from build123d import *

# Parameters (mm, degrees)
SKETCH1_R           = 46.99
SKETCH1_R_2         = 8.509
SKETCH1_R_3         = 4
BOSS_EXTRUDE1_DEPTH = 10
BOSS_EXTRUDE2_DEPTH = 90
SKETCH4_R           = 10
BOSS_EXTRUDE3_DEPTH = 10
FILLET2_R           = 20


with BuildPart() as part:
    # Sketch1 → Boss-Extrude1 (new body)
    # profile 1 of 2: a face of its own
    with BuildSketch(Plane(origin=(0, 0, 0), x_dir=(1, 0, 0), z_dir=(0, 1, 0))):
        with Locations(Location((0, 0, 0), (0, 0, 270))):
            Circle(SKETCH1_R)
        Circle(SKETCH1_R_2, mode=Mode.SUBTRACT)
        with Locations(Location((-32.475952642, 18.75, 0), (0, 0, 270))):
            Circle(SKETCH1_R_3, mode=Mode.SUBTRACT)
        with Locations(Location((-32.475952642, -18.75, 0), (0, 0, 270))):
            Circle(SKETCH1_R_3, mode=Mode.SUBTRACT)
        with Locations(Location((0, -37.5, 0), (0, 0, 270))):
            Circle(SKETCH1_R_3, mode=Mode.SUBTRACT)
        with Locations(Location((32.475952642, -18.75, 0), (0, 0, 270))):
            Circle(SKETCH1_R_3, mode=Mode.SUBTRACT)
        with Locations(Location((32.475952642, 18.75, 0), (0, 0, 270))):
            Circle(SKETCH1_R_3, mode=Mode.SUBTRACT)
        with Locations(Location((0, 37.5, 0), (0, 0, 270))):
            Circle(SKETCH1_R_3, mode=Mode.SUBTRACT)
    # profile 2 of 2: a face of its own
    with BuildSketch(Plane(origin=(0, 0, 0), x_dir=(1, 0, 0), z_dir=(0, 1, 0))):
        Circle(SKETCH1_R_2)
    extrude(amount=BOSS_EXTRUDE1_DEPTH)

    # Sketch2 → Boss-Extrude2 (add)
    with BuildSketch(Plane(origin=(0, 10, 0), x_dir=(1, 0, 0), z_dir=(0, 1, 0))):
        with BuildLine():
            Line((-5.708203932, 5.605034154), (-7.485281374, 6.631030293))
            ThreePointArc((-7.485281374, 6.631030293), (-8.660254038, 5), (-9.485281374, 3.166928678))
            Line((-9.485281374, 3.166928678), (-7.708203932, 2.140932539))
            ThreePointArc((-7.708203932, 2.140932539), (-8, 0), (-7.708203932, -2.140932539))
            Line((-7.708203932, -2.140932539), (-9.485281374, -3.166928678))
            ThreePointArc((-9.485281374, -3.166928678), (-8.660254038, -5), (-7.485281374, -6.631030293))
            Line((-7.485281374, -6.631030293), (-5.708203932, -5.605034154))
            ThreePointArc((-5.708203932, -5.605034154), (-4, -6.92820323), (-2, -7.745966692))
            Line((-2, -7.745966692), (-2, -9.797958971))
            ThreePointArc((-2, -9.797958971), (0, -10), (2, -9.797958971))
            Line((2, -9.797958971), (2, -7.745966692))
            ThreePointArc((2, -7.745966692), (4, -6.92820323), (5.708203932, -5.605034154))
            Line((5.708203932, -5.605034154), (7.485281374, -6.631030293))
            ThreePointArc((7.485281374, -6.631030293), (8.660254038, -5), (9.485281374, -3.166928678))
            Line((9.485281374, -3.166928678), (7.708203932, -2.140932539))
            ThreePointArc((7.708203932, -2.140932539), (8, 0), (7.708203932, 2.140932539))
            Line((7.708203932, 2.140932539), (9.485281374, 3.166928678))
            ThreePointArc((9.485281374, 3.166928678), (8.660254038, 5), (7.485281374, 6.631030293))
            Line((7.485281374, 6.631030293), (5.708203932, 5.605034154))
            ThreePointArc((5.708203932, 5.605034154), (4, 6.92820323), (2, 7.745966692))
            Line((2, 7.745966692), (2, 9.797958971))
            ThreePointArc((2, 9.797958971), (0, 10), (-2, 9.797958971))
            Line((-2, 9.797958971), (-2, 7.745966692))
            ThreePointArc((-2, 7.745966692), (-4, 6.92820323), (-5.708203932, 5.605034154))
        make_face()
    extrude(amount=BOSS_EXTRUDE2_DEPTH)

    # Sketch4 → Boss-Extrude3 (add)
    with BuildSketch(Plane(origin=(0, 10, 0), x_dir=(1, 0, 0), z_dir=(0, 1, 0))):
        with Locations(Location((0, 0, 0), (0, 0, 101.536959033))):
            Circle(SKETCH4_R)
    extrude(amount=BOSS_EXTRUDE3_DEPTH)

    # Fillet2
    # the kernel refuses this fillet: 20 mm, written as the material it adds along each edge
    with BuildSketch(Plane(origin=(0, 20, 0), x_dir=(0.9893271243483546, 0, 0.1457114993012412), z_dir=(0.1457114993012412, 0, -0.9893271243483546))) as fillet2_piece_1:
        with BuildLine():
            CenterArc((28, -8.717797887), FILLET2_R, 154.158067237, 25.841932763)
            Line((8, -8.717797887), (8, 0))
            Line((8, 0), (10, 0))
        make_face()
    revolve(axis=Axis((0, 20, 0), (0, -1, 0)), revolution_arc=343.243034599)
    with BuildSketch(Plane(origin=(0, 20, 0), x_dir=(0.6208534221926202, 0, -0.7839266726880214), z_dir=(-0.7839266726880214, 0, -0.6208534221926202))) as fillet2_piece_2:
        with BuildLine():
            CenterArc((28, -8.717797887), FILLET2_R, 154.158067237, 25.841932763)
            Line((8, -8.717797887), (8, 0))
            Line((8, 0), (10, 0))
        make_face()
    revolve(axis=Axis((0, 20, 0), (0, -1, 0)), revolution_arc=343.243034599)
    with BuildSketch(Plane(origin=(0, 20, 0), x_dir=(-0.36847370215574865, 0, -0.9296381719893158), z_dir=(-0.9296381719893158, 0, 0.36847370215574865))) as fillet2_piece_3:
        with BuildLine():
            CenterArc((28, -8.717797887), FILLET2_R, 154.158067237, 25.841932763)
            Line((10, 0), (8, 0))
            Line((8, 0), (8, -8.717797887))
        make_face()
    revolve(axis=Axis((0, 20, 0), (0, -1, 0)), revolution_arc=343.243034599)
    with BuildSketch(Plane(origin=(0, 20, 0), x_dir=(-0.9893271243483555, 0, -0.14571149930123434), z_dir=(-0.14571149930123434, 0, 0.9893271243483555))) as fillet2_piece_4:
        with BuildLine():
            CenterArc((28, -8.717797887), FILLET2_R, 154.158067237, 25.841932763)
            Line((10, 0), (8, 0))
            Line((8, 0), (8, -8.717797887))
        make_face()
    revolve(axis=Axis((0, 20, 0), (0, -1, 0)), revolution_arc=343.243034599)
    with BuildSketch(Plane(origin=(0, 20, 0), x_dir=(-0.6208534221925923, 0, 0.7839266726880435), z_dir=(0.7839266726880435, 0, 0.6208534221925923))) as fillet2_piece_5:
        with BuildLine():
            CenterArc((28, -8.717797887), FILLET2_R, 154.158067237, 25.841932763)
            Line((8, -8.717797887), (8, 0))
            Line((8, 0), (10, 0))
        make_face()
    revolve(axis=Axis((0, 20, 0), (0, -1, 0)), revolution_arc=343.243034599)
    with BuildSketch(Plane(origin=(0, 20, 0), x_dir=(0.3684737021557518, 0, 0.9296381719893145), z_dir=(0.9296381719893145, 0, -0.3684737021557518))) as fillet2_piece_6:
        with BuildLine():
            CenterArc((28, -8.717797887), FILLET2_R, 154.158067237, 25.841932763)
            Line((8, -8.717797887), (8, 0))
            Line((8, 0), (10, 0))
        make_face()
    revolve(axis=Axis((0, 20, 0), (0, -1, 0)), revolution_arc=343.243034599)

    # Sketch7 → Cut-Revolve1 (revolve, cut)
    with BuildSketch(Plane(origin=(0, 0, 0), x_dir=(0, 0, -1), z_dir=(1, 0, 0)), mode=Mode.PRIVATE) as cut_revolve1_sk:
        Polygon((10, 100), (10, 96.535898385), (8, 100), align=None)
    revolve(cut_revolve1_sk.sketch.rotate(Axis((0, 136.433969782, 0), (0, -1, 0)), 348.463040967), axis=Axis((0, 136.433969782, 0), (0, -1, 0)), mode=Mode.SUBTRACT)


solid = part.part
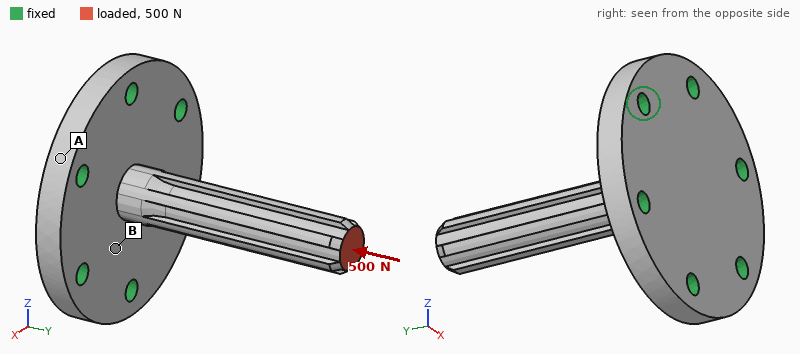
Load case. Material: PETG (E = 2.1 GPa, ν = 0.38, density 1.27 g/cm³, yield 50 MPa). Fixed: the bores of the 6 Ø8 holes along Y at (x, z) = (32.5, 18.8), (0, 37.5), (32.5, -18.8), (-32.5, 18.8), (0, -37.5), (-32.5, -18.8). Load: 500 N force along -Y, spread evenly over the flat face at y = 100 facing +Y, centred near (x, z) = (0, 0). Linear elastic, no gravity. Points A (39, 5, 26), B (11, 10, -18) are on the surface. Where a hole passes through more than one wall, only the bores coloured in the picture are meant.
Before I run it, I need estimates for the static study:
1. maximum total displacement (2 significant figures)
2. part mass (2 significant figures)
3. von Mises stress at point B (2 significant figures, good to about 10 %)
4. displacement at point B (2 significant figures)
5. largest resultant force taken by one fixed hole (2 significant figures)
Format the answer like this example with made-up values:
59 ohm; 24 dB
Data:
0.14 mm; 110 g; 1.00 MPa; 0.031 mm; 86 N
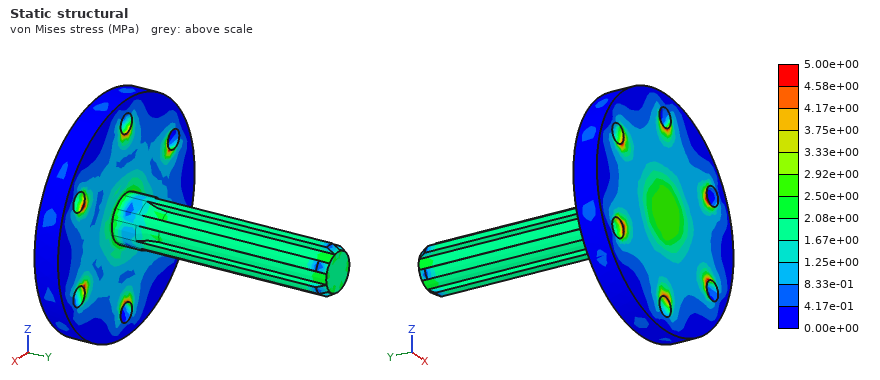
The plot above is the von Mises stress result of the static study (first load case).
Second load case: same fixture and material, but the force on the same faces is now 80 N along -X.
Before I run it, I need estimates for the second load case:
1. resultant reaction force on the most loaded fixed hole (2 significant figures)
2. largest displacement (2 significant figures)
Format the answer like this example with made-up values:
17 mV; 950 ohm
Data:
80 N; 2.0 mm
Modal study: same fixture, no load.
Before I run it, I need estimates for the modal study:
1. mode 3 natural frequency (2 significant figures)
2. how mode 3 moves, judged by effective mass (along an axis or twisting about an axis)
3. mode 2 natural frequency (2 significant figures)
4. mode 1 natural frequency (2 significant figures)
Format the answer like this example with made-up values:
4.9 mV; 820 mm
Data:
2000 Hz; along Y; 380 Hz; 380 Hz
